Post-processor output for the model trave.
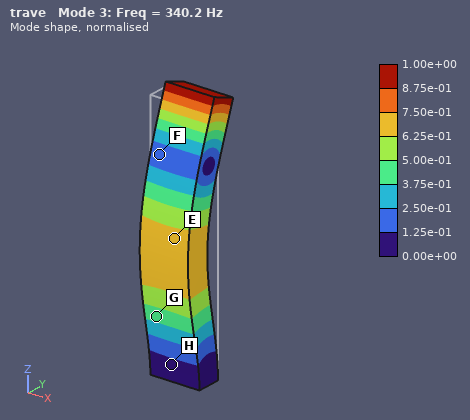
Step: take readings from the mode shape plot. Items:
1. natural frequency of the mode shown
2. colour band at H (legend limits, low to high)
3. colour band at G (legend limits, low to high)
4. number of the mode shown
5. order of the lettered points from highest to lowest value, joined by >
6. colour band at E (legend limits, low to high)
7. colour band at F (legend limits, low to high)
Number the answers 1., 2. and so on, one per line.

1. 340.2 Hz
2. 0.00e+00 to 1.25e-01
3. 3.75e-01 to 5.00e-01
4. 3
5. E > G > F > H
6. 6.25e-01 to 7.50e-01
7. 1.25e-01 to 2.50e-01
